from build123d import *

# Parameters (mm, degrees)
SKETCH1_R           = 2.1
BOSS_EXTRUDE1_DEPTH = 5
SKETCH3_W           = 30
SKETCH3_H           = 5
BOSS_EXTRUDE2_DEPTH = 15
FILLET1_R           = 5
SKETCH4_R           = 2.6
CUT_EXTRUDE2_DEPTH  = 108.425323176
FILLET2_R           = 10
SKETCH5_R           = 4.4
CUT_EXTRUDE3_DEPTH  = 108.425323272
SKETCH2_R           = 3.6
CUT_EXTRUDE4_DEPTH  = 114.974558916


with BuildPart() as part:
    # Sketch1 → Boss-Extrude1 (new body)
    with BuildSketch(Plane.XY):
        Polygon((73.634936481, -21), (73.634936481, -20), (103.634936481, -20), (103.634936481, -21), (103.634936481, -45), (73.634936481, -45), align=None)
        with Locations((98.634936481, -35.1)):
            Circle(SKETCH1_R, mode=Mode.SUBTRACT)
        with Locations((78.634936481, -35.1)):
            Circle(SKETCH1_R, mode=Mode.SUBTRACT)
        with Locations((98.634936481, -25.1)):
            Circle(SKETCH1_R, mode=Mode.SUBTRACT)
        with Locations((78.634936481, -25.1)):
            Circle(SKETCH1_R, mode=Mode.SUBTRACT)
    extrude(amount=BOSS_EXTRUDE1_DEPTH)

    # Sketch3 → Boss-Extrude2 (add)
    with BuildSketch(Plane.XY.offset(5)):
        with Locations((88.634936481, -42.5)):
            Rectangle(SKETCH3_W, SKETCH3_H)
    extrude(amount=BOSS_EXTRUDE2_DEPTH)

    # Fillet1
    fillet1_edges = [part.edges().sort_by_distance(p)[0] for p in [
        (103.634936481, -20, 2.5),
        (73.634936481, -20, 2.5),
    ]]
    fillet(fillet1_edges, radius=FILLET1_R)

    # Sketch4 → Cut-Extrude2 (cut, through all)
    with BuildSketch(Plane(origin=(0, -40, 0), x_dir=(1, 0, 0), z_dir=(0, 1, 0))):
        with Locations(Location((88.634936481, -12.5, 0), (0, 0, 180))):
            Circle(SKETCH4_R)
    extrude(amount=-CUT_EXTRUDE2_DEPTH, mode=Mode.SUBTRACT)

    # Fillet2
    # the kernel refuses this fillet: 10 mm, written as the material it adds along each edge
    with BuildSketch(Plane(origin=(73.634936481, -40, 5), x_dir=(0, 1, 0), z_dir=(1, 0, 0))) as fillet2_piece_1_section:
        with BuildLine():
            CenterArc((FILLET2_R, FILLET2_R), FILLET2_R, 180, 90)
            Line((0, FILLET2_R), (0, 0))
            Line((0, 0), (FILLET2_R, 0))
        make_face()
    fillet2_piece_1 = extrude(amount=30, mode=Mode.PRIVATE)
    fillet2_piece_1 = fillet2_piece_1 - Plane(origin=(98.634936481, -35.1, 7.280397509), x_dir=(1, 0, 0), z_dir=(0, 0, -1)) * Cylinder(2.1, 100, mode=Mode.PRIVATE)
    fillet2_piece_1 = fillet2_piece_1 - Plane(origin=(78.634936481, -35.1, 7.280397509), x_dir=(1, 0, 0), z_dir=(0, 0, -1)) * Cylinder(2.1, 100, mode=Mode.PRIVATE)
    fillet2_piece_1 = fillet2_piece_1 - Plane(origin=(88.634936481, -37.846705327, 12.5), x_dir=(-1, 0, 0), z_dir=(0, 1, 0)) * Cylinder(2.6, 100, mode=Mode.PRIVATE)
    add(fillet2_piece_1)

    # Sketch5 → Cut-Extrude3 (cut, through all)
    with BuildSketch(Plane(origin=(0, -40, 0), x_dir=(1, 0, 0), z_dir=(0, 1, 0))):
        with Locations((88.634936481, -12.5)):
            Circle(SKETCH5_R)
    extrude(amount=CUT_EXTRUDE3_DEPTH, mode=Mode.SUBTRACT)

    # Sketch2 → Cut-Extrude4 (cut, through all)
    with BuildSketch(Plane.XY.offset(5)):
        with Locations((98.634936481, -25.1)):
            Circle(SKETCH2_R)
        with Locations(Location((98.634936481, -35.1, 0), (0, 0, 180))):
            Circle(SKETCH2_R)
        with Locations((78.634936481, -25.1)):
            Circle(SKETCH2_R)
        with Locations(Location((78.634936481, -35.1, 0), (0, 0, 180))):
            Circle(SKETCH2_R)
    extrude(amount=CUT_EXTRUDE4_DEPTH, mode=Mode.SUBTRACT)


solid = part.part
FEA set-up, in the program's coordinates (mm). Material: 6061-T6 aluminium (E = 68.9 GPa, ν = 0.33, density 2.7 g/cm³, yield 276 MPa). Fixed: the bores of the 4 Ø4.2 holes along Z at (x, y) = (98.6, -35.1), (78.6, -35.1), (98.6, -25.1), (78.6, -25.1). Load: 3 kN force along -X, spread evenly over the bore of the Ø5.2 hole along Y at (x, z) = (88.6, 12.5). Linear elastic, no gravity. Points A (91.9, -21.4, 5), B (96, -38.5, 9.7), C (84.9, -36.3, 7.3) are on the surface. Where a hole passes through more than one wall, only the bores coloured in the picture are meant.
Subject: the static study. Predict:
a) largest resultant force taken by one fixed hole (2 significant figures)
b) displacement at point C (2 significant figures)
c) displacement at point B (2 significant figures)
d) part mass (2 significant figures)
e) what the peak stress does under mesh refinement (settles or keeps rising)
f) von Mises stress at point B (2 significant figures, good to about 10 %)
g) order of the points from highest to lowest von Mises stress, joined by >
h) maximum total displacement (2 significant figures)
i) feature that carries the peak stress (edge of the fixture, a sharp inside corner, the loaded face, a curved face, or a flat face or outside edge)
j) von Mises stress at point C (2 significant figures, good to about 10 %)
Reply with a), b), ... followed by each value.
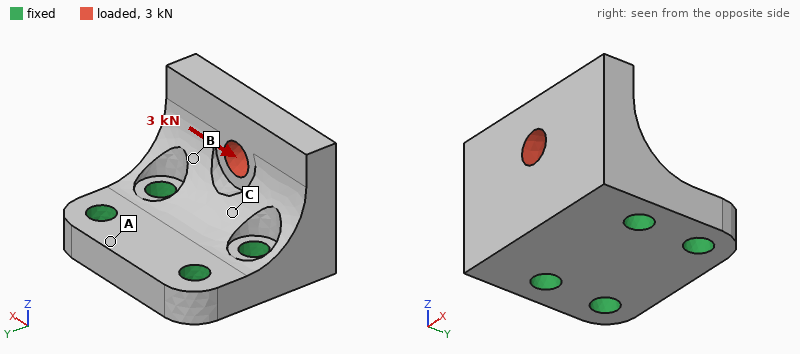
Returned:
a) 2.1 kN
b) 4.8 µm
c) 11 µm
d) 16 g
e) keeps rising
f) 41 MPa
g) C > B > A
h) 26 µm
i) edge of the fixture
j) 52 MPa
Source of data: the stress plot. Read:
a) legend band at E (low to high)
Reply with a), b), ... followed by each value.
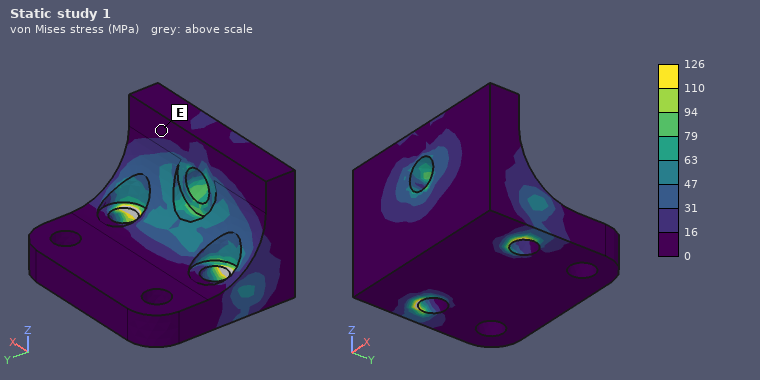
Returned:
a) 0 to 16 MPa
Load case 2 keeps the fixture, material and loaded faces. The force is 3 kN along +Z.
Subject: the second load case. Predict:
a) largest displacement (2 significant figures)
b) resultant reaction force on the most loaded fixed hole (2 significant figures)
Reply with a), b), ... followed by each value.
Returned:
a) 57 µm
b) 1.8 kN
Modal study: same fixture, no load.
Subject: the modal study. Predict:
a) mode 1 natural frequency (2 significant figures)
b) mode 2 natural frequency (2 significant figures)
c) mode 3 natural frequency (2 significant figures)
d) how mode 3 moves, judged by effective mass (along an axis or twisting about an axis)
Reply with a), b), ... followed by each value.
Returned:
a) 12 kHz
b) 20 kHz
c) 28 kHz
d) along X
